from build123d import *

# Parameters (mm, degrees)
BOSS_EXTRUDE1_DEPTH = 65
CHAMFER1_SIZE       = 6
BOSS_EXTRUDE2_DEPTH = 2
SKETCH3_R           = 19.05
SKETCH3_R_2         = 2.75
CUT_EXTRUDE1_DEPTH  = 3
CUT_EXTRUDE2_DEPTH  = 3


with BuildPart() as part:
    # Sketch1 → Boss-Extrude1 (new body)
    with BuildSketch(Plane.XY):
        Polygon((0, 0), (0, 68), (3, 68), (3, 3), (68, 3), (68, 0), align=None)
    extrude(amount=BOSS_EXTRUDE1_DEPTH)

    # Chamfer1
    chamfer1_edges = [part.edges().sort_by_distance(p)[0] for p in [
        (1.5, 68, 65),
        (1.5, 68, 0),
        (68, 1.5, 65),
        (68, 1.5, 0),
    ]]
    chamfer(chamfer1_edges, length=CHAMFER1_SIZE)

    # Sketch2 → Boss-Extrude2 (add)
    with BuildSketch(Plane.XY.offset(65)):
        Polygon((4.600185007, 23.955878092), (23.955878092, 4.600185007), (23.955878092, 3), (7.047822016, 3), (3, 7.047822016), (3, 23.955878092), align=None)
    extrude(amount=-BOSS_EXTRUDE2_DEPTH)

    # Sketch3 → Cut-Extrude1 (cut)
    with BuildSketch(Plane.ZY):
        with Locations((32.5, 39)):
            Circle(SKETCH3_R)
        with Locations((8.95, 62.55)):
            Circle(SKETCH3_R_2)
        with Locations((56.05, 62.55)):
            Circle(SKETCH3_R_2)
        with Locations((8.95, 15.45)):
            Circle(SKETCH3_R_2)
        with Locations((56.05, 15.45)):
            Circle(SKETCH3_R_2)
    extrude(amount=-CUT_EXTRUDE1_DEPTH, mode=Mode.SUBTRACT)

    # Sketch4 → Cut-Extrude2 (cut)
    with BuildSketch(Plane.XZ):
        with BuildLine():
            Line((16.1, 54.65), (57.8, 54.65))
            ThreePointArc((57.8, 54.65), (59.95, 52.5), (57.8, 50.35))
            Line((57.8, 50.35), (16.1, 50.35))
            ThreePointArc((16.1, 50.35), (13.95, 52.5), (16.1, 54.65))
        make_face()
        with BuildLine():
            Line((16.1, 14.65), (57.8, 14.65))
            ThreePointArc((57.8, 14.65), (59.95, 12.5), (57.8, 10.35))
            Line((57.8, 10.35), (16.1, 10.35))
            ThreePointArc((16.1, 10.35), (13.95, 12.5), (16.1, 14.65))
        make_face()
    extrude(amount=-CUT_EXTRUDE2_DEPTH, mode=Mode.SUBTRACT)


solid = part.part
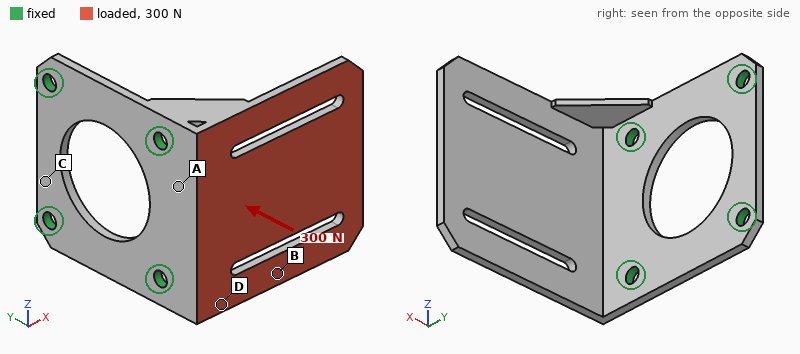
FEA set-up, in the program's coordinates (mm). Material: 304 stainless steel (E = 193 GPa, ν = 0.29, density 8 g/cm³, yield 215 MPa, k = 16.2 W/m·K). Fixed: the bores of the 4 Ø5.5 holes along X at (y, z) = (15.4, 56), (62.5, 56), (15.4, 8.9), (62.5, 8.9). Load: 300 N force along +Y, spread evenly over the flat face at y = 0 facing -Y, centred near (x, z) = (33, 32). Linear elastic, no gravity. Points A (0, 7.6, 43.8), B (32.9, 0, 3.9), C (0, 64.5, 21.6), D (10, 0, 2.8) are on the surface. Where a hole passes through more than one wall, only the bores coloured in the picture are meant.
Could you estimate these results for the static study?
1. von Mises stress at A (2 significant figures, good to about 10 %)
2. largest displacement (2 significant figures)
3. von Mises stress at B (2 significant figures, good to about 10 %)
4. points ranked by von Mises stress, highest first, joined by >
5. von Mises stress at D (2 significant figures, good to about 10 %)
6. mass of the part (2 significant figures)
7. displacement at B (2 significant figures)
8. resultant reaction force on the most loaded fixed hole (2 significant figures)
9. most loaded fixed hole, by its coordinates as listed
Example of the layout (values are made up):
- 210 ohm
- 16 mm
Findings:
- 44 MPa
- 0.52 mm
- 24 MPa
- D > A > B > C
- 61 MPa
- 170 g
- 0.20 mm
- 180 N
- (15.4, 8.9)
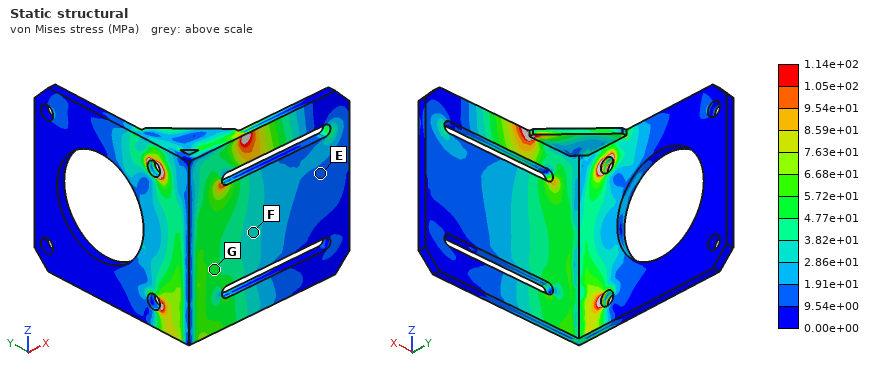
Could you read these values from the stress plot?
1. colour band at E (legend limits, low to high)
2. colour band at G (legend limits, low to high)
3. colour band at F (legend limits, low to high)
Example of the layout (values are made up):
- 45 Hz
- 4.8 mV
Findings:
- 9.54e+00 to 1.91e+01 MPa
- 4.77e+01 to 5.72e+01 MPa
- 2.86e+01 to 3.82e+01 MPa
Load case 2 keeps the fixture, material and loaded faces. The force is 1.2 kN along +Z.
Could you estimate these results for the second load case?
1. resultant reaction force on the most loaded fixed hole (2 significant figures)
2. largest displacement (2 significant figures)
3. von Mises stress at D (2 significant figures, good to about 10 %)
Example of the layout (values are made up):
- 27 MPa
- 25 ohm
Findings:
- 1.0 kN
- 0.11 mm
- 34 MPa
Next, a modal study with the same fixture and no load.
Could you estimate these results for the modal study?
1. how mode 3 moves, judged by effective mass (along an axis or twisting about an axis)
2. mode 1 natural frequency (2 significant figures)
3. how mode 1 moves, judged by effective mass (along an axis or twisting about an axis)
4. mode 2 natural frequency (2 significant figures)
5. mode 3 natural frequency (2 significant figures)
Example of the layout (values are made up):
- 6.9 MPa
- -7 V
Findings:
- along Z
- 500 Hz
- along Y
- 1400 Hz
- 2200 Hz
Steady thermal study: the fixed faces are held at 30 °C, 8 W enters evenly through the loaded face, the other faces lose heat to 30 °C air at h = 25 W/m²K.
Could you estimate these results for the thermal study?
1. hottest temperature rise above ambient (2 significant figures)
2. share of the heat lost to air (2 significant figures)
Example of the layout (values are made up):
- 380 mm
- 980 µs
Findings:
- 45 K
- 65 %
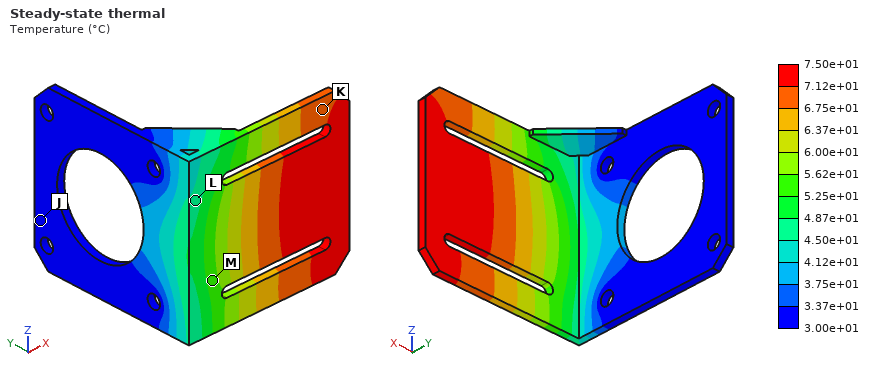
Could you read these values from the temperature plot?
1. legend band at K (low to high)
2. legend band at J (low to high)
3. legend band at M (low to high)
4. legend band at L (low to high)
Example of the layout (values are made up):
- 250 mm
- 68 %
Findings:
- 6.75e+01 to 7.12e+01 °C
- 3.00e+01 to 3.37e+01 °C
- 5.25e+01 to 5.62e+01 °C
- 4.50e+01 to 4.87e+01 °C
